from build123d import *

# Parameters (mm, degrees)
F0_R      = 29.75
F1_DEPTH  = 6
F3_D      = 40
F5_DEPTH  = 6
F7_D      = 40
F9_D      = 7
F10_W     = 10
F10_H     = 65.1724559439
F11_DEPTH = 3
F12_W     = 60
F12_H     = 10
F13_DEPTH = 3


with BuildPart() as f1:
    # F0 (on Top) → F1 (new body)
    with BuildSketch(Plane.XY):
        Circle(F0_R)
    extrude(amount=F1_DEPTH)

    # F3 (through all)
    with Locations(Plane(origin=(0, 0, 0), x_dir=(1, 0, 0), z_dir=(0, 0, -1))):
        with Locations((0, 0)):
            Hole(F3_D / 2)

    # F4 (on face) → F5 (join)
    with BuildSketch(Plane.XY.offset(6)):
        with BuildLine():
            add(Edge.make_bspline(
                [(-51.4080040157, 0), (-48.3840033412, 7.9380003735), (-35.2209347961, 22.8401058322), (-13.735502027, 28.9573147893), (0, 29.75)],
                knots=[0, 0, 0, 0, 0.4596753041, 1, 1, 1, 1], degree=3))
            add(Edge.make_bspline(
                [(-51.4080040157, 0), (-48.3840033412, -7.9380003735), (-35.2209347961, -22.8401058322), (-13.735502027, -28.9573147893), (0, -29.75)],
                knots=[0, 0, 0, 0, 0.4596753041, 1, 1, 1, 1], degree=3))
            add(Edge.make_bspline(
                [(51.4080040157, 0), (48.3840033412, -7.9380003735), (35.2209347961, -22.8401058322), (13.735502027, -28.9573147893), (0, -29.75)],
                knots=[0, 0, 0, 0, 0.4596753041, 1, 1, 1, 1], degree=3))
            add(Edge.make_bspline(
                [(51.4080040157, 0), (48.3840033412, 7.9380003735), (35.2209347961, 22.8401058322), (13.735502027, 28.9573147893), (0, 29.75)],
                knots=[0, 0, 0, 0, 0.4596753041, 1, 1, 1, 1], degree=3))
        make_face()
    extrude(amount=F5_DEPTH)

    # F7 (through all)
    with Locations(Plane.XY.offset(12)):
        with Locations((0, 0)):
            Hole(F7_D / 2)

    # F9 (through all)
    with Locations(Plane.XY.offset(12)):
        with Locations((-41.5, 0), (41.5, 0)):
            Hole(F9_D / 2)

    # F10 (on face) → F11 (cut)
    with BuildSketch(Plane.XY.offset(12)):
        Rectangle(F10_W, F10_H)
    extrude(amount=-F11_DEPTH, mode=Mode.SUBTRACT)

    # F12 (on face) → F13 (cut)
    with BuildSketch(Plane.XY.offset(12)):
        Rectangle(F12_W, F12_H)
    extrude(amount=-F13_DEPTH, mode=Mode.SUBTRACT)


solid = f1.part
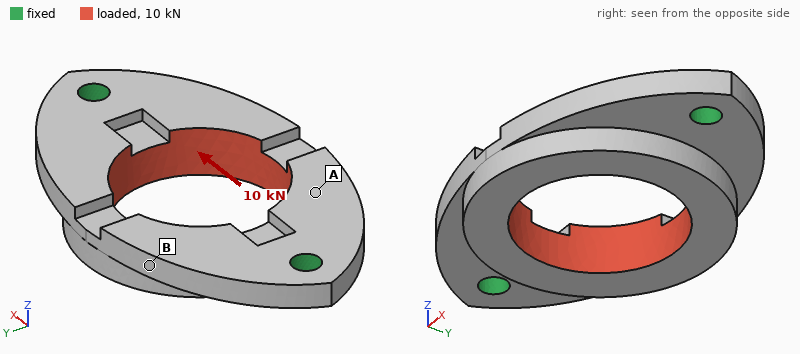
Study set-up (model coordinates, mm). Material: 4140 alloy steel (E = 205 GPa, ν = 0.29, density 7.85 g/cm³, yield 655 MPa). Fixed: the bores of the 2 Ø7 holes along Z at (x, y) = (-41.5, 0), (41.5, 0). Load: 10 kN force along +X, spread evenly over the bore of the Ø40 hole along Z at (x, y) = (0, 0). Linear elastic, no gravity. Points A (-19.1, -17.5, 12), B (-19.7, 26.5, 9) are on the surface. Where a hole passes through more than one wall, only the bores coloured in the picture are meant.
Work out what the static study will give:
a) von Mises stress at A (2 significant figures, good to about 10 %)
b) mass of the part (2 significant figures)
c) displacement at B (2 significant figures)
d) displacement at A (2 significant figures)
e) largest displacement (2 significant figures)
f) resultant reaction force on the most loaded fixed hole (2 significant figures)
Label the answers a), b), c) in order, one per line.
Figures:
a) 23 MPa
b) 210 g
c) 5.5 µm
d) 4.8 µm
e) 6.6 µm
f) 5.0 kN
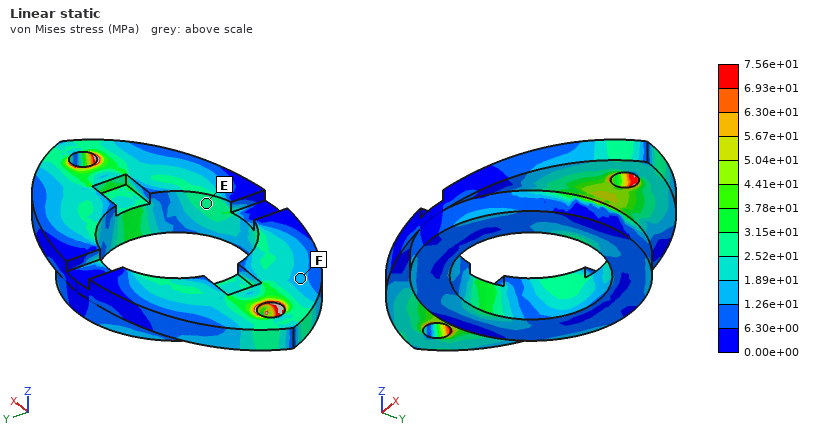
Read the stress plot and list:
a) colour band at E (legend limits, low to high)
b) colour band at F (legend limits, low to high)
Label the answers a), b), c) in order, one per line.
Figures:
a) 2.52e+01 to 3.15e+01 MPa
b) 1.26e+01 to 1.89e+01 MPa
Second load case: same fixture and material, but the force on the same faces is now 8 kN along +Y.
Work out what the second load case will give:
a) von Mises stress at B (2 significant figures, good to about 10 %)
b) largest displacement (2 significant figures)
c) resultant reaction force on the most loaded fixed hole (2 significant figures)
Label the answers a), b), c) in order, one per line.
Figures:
a) 26 MPa
b) 42 µm
c) 4.0 kN
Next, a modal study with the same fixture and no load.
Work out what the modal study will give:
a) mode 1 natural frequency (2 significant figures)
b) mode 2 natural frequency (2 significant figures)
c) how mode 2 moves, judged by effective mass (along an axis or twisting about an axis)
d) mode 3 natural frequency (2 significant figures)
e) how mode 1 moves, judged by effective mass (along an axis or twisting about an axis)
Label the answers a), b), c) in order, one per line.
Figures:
a) 3200 Hz
b) 4300 Hz
c) along Z
d) 10 kHz
e) twisting about X
